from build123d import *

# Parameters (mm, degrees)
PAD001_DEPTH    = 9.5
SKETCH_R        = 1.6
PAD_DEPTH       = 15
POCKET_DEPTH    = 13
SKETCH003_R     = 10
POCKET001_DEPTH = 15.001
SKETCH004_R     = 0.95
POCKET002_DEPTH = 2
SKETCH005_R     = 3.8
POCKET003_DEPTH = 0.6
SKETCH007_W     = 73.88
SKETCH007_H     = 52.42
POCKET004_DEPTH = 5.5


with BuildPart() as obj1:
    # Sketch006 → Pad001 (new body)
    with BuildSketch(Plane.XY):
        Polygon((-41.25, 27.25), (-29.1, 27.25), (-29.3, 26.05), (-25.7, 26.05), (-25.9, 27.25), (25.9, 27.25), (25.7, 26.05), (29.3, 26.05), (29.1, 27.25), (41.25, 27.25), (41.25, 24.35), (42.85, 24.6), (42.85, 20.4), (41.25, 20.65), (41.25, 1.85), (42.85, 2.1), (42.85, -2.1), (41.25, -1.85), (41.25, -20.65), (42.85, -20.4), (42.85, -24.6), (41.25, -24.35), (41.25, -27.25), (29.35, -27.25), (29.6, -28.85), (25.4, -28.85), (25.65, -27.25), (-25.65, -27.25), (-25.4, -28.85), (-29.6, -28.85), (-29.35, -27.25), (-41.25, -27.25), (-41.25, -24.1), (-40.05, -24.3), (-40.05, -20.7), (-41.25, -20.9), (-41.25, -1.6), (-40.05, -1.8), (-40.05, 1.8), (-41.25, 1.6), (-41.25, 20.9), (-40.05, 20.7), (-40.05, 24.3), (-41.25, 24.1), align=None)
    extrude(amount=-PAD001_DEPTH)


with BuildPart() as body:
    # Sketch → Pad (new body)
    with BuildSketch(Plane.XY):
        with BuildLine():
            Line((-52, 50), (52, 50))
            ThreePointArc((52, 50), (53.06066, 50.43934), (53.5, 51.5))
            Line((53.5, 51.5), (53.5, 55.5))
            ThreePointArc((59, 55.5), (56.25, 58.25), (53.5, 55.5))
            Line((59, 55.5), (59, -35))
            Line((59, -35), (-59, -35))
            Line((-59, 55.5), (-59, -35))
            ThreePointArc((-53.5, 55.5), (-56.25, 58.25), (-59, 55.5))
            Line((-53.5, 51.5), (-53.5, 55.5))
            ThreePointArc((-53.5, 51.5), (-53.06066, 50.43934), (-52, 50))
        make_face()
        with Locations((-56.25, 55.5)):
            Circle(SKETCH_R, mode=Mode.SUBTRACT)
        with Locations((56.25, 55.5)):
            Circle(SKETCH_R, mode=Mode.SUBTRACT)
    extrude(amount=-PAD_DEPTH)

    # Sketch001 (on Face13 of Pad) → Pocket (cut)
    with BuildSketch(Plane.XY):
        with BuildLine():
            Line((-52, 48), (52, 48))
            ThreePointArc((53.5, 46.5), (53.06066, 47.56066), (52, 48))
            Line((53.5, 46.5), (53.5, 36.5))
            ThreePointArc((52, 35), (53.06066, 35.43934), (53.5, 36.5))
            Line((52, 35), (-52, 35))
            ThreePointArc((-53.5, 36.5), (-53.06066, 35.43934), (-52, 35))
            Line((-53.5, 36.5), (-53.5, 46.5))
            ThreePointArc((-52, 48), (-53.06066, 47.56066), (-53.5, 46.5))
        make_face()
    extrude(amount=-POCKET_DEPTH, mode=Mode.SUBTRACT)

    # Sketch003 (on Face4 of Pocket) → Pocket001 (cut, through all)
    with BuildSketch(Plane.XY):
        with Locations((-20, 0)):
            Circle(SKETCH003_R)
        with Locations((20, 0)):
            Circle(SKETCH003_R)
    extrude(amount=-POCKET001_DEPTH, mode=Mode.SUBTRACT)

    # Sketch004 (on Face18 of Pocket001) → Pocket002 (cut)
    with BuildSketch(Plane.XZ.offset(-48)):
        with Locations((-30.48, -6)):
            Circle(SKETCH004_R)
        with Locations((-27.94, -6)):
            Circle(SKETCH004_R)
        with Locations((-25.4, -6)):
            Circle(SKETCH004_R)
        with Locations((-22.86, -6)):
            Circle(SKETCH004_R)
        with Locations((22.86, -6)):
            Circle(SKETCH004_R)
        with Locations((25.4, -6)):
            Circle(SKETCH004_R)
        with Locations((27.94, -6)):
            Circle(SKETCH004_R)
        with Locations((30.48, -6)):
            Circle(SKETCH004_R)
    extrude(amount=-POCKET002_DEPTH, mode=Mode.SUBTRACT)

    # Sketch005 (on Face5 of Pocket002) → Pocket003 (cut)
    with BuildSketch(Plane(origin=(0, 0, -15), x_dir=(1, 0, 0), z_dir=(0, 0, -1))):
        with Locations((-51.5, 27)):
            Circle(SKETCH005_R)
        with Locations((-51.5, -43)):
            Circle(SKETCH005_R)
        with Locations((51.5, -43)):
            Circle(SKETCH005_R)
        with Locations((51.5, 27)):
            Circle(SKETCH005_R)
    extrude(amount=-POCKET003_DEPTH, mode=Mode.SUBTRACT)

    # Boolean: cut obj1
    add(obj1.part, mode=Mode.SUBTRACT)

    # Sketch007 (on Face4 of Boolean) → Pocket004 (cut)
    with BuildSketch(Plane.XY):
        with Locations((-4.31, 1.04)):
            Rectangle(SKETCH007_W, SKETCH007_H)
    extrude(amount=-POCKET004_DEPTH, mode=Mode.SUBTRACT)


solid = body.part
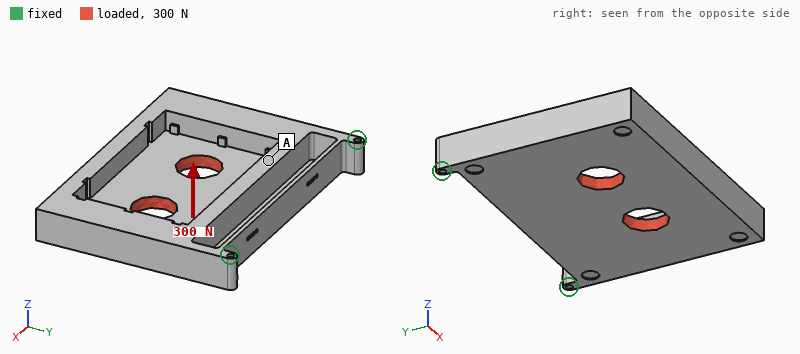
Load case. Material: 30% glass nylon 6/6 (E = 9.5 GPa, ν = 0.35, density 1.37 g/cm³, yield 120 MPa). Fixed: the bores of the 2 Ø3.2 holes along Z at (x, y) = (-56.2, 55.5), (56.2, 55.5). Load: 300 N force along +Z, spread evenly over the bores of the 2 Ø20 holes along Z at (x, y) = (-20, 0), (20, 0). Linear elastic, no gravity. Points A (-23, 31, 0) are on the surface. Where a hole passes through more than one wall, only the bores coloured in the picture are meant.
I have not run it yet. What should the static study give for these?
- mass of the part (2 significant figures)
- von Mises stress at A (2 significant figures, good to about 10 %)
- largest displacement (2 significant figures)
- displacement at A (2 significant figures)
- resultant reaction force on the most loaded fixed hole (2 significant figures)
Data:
120 g
5.7 MPa
0.89 mm
0.22 mm
170 N
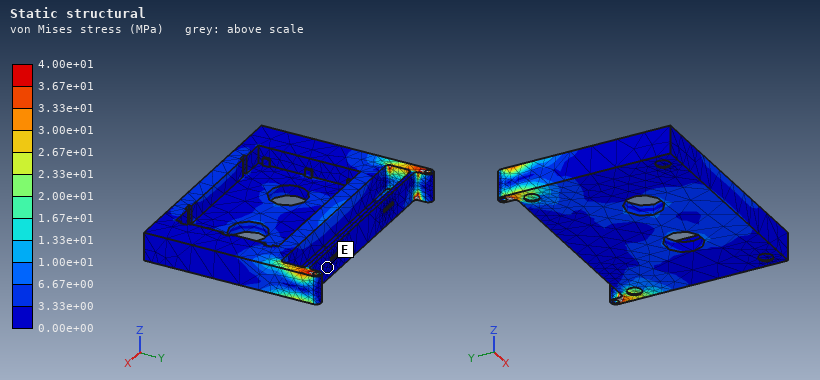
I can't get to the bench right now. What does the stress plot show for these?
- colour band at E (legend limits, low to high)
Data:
0.00e+00 to 3.33e+00 MPa
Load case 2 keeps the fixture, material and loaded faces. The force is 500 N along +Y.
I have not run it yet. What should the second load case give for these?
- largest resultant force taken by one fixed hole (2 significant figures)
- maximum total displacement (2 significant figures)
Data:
260 N
0.13 mm
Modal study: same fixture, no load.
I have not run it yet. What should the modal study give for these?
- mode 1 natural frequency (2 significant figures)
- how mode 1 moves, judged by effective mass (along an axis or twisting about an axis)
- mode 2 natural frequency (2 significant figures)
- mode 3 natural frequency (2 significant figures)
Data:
340 Hz
along Z
750 Hz
1600 Hz
